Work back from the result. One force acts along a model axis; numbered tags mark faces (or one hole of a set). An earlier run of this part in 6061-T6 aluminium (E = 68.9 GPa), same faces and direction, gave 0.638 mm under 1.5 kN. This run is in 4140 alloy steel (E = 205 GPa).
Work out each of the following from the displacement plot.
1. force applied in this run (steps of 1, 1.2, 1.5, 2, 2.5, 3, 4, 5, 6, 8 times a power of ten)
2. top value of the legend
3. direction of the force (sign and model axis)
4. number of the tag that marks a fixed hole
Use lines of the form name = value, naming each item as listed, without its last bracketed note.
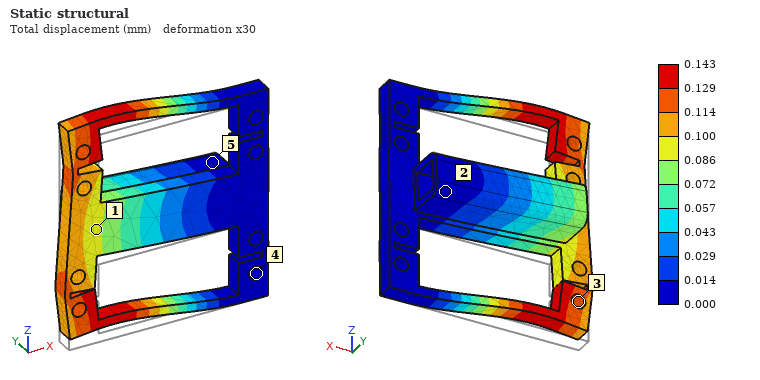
force applied in this run = 1 kN
top value of the legend = 0.143 mm
direction of the force = +Z
number of the tag that marks a fixed hole = 4
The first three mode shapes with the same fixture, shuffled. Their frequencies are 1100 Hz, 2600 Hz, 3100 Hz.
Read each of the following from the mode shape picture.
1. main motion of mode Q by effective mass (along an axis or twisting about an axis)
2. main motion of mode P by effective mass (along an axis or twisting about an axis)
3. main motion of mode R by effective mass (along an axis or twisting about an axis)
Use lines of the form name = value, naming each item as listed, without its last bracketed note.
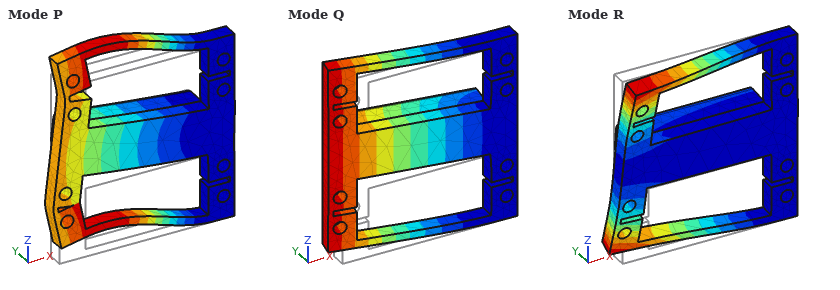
main motion of mode Q by effective mass = along Y
main motion of mode P by effective mass = along Z
main motion of mode R by effective mass = twisting about X
